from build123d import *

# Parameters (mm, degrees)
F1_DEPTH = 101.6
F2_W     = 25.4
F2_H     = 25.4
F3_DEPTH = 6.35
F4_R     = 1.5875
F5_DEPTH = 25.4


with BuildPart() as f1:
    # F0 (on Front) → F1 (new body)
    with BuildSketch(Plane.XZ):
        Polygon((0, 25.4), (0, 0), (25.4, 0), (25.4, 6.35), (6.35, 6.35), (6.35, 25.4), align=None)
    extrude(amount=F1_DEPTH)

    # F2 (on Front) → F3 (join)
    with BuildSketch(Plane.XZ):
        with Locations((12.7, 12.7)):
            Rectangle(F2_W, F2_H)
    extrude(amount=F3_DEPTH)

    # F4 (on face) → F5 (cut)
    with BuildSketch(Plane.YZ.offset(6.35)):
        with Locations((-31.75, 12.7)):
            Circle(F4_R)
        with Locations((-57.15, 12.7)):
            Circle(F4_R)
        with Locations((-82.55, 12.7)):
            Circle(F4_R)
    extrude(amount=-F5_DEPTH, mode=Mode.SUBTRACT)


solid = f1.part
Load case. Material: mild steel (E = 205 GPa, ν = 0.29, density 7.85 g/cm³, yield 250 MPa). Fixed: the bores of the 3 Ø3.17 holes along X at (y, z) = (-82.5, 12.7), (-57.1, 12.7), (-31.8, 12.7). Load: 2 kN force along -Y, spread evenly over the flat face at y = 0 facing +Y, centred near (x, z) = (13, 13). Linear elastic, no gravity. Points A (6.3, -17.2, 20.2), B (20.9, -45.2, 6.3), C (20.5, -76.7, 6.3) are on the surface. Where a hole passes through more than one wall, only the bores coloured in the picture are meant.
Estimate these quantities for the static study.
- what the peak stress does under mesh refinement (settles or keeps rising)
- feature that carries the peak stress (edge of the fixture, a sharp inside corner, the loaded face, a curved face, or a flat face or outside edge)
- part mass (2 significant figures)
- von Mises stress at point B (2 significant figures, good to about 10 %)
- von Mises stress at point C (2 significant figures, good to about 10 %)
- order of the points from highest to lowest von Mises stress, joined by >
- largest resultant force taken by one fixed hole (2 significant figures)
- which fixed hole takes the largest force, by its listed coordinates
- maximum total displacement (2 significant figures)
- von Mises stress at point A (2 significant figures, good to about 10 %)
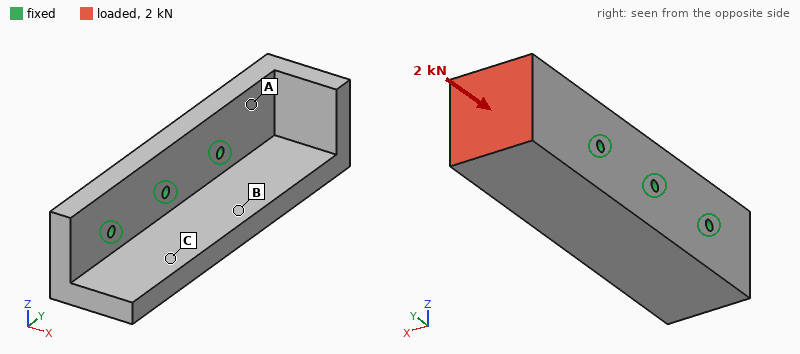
keeps rising
edge of the fixture
240 g
11 MPa
3.7 MPa
A > B > C
1.2 kN
(-31.8, 12.7)
25 µm
26 MPa
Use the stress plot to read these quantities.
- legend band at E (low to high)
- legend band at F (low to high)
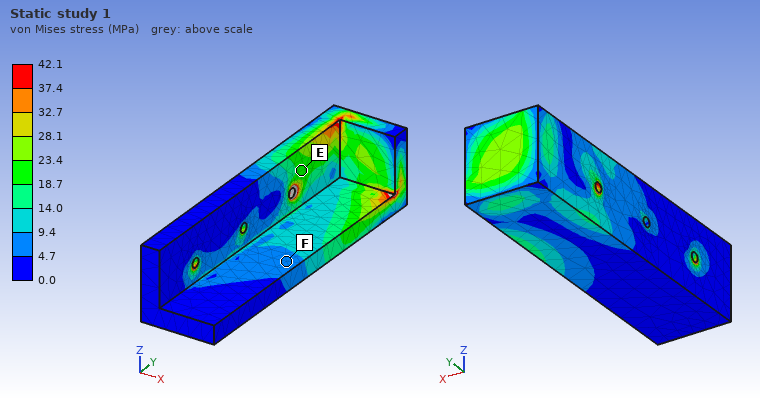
18.7 to 23.4 MPa
4.7 to 9.4 MPa
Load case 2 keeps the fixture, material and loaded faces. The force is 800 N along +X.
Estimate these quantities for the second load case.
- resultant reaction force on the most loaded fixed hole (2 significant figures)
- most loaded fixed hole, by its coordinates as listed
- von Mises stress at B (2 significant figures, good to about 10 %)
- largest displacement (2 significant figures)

1.4 kN
(-31.8, 12.7)
11 MPa
23 µm
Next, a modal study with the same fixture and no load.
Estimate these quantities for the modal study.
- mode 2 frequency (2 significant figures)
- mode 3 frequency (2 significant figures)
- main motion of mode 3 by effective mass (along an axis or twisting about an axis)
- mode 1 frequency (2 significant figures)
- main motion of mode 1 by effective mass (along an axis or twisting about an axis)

5100 Hz
6100 Hz
along X
4000 Hz
along Z
